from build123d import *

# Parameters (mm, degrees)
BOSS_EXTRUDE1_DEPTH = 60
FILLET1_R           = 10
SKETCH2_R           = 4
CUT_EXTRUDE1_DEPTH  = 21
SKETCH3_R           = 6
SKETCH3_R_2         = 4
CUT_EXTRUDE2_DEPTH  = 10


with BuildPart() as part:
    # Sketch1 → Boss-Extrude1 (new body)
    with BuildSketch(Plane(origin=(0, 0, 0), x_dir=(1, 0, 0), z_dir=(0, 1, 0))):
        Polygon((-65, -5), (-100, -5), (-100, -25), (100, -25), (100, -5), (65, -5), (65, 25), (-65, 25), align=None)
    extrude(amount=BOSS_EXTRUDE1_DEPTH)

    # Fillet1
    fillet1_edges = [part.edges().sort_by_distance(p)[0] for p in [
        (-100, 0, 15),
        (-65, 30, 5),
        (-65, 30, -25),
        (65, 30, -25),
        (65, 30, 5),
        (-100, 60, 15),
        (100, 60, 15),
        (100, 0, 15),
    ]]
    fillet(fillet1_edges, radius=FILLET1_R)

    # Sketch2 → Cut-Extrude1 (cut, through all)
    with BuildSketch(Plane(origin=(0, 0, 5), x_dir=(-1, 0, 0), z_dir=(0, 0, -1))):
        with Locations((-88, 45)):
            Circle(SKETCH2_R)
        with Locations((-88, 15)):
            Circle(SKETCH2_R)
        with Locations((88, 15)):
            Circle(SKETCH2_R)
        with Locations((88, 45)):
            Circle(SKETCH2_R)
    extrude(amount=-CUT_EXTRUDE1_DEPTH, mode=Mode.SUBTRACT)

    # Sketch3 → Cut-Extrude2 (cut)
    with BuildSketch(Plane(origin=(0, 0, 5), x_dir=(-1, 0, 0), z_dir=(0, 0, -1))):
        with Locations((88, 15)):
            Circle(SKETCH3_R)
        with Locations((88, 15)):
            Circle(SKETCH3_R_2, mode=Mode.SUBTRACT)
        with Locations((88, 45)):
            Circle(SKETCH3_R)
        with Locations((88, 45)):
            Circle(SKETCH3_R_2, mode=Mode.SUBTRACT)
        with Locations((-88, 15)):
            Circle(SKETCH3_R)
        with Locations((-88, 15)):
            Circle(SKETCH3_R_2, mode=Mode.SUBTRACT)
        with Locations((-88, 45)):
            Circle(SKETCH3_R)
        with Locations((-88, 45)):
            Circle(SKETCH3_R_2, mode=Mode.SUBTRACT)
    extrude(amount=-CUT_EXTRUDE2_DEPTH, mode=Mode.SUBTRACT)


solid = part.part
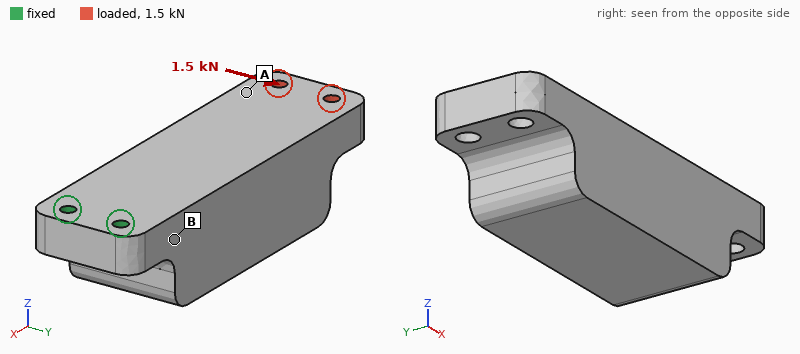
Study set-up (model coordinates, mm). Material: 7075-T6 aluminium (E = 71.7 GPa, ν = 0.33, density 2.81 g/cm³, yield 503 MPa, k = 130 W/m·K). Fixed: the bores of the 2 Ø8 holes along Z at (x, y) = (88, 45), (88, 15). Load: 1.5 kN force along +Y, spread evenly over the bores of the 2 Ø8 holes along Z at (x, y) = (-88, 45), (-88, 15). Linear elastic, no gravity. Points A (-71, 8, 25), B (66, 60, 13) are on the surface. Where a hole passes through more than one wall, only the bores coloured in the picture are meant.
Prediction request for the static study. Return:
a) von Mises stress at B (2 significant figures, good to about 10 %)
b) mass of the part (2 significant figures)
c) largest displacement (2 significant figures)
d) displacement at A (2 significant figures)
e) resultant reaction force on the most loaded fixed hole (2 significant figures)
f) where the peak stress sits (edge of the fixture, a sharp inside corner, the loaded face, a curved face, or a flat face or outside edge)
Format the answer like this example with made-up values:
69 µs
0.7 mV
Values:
17 MPa
1.3 kg
0.15 mm
0.12 mm
7.5 kN
edge of the fixture
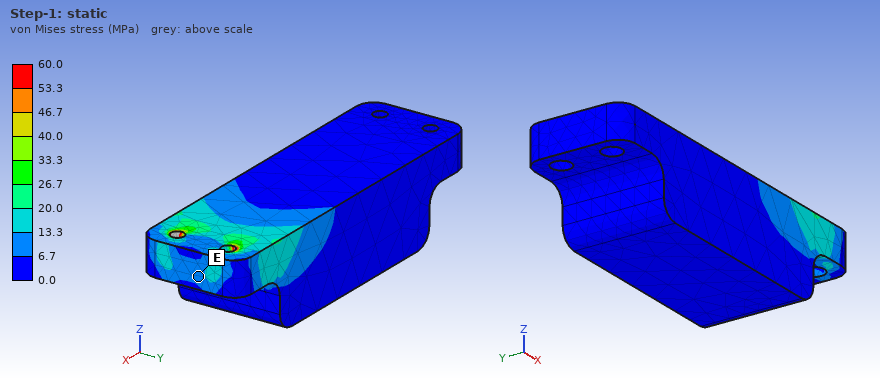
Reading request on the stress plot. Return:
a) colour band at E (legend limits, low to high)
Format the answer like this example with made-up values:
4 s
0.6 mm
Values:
6.7 to 13.3 MPa
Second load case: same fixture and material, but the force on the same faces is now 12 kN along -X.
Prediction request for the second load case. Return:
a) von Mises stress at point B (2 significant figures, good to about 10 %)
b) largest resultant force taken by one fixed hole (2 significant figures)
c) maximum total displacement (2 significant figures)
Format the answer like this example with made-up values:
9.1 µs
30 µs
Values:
7.6 MPa
6.0 kN
0.18 mm
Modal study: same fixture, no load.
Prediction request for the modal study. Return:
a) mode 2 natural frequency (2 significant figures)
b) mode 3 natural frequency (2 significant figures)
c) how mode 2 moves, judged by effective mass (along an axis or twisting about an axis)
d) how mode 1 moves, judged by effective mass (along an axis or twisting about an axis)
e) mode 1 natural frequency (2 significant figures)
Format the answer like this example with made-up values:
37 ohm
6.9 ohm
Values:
900 Hz
2200 Hz
along Y
along Z
330 Hz
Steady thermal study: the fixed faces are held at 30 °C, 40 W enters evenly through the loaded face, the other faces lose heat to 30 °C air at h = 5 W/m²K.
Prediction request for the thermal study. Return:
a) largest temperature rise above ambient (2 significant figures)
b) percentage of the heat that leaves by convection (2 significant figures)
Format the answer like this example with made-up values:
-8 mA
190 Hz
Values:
31 K
8.2 %
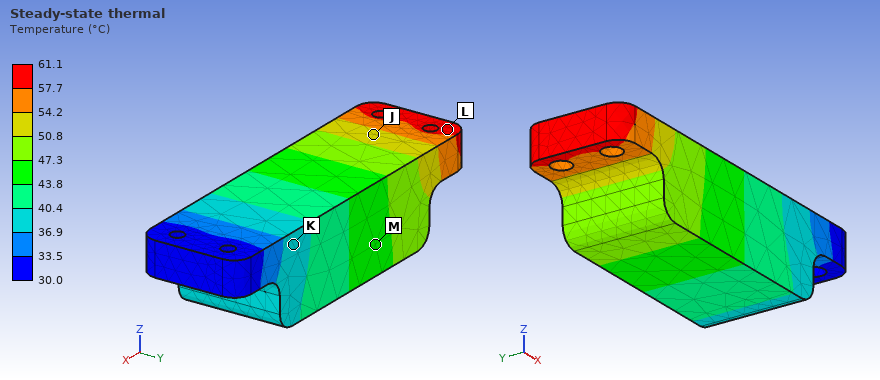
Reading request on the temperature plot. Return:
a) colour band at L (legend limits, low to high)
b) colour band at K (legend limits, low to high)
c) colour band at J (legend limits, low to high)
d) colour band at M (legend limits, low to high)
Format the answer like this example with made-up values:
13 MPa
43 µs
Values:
57.7 to 61.1 °C
36.9 to 40.4 °C
50.8 to 54.2 °C
43.8 to 47.3 °C
